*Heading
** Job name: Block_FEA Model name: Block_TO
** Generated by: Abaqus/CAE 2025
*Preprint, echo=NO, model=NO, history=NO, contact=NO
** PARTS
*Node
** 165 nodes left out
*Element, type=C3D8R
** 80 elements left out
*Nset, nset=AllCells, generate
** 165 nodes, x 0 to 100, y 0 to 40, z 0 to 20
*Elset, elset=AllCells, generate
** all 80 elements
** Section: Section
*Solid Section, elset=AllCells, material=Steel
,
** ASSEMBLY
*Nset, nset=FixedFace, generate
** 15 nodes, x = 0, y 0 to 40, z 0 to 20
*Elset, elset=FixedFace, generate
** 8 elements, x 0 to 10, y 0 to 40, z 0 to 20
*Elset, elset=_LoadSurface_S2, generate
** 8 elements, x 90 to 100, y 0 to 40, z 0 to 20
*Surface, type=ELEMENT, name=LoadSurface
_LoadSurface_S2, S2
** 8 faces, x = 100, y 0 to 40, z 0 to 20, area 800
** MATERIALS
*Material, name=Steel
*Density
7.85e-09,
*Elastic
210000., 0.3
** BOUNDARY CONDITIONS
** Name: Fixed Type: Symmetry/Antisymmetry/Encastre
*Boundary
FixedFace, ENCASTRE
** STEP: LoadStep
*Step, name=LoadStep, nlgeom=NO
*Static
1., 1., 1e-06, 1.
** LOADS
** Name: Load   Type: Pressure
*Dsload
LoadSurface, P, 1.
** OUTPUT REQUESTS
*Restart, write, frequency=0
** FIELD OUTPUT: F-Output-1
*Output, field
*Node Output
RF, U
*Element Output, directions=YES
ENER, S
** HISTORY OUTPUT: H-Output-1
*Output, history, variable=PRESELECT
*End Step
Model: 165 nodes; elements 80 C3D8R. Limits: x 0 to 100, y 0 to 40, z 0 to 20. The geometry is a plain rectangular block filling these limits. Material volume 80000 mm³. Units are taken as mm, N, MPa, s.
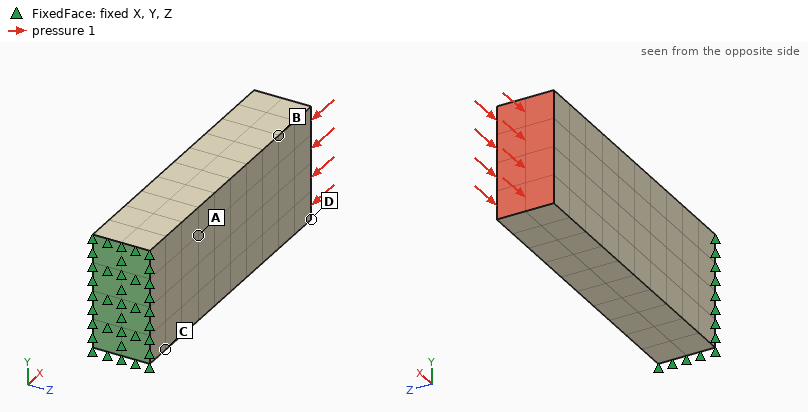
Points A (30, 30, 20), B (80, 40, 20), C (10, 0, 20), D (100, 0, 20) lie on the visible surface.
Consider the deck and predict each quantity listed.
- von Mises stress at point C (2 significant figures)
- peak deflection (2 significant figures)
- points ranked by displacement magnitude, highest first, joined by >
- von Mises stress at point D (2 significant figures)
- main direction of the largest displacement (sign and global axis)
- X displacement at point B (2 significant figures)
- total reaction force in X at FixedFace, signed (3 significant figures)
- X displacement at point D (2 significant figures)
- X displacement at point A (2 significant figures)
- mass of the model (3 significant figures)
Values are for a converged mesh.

0.96 MPa
4.7e-04 mm
D > B > A > C
1.0 MPa
-X
-3.8e-04 mm
800 N
-4.7e-04 mm
-1.4e-04 mm
0.628 kg
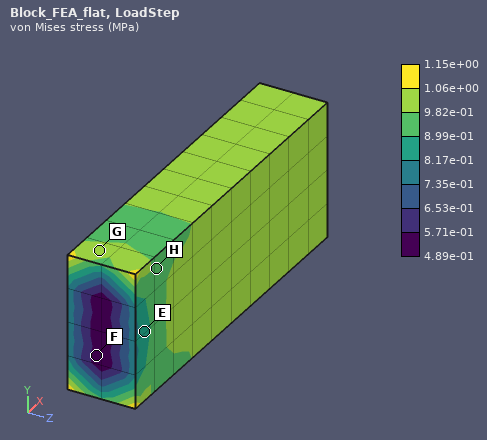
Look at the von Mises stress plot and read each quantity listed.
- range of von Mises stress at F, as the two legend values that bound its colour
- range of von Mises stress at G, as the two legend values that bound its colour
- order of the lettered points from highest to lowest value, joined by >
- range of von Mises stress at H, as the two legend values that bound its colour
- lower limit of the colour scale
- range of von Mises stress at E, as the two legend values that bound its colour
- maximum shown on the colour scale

4.89e-01 to 5.71e-01 MPa
9.82e-01 to 1.06e+00 MPa
G > H > E > F
8.99e-01 to 9.82e-01 MPa
4.89e-01 MPa
8.17e-01 to 8.99e-01 MPa
1.15e+00 MPa
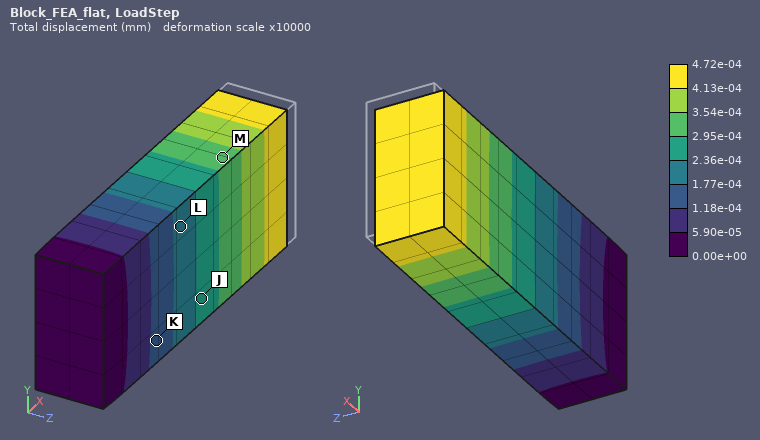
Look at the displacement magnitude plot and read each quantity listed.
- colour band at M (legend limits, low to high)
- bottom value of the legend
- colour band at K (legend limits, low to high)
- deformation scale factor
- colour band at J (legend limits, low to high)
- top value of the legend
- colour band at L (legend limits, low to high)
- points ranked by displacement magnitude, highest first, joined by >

2.95e-04 to 3.54e-04 mm
0.00e+00 mm
1.18e-04 to 1.77e-04 mm
10000
2.36e-04 to 2.95e-04 mm
4.72e-04 mm
1.77e-04 to 2.36e-04 mm
M > J > L > K
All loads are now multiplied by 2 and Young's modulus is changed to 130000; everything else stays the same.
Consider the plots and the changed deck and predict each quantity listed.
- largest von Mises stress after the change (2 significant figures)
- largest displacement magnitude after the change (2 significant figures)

2.3 MPa
0.0015 mm
